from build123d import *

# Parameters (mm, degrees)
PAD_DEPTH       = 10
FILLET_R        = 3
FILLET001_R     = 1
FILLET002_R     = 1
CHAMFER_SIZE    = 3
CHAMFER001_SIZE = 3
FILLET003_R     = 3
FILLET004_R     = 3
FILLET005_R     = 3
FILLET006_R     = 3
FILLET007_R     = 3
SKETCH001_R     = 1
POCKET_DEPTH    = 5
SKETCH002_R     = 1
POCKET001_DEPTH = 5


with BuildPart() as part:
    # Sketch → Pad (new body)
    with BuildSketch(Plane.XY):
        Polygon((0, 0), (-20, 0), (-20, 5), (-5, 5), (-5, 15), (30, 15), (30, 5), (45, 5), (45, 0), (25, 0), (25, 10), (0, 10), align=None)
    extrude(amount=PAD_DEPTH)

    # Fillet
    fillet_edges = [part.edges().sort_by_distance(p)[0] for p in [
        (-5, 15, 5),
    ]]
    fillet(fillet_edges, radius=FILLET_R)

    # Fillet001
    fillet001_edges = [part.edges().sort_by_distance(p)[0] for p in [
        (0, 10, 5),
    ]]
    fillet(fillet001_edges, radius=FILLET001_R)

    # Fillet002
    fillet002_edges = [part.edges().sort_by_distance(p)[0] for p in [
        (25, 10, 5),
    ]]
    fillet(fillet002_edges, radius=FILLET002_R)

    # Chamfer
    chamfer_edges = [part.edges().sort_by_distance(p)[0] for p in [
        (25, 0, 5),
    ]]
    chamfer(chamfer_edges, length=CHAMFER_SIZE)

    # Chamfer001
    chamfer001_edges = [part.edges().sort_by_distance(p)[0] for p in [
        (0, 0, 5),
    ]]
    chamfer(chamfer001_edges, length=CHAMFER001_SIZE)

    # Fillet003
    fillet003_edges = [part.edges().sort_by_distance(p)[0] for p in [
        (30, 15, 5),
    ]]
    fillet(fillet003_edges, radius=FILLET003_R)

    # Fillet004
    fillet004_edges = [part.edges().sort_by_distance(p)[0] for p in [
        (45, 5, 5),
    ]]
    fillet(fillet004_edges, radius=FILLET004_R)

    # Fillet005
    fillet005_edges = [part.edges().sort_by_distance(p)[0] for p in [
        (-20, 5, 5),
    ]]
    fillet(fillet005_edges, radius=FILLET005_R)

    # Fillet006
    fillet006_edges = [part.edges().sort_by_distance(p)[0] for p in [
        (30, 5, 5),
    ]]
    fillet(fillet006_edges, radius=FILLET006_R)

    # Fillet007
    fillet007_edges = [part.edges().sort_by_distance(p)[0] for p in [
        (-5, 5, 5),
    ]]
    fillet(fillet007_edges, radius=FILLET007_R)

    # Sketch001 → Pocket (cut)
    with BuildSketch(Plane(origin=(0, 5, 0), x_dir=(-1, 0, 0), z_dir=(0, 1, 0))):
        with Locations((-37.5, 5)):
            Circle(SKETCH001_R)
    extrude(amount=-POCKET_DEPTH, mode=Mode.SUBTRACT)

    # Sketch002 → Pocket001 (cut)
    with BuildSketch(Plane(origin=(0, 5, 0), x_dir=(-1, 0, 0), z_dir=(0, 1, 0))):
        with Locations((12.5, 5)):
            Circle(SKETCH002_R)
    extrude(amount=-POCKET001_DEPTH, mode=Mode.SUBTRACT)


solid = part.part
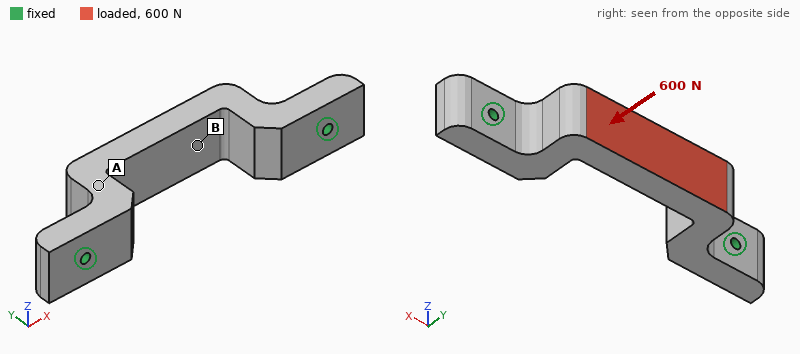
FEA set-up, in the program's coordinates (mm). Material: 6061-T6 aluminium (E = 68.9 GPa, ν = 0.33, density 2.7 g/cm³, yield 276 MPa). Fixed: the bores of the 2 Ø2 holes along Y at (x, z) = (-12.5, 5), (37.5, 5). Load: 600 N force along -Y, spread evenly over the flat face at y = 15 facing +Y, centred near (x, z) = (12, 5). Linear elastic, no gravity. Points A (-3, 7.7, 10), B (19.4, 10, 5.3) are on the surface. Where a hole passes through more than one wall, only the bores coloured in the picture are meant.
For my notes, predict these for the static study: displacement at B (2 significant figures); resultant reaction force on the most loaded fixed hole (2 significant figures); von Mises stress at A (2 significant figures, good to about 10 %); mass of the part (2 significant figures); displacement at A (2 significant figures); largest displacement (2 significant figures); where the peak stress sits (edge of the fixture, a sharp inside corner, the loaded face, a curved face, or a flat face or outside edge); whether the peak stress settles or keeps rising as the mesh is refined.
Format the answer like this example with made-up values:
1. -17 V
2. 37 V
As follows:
1. 12 µm
2. 440 N
3. 18 MPa
4. 11 g
5. 6.0 µm
6. 15 µm
7. edge of the fixture
8. keeps rising
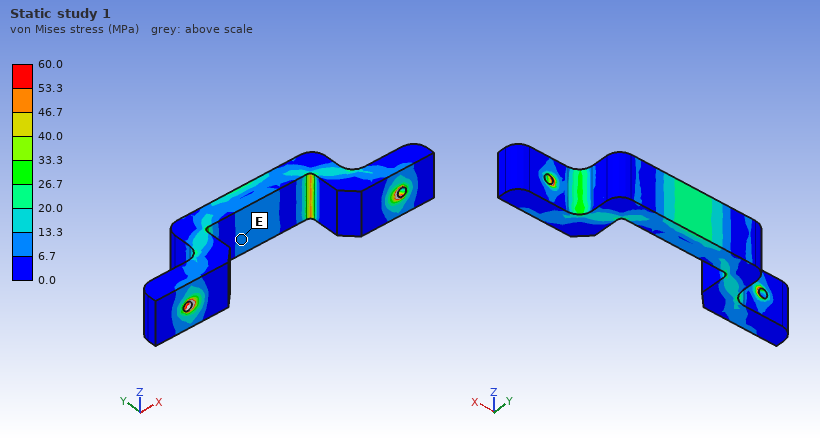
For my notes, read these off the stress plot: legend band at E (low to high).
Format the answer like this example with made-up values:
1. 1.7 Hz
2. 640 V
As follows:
1. 6.7 to 13.3 MPa
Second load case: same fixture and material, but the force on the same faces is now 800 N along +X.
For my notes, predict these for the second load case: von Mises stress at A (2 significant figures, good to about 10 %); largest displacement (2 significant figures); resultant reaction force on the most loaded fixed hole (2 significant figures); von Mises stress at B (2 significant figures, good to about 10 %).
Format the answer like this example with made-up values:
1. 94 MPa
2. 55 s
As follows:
1. 24 MPa
2. 14 µm
3. 440 N
4. 24 MPa
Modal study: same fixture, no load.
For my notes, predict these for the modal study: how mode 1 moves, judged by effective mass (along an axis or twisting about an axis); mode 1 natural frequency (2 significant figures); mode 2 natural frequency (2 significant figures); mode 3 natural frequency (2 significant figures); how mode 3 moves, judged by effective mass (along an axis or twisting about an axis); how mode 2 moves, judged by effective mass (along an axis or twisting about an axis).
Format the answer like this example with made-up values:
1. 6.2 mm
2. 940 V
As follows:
1. along Z
2. 6900 Hz
3. 14 kHz
4. 16 kHz
5. along Y
6. along X
